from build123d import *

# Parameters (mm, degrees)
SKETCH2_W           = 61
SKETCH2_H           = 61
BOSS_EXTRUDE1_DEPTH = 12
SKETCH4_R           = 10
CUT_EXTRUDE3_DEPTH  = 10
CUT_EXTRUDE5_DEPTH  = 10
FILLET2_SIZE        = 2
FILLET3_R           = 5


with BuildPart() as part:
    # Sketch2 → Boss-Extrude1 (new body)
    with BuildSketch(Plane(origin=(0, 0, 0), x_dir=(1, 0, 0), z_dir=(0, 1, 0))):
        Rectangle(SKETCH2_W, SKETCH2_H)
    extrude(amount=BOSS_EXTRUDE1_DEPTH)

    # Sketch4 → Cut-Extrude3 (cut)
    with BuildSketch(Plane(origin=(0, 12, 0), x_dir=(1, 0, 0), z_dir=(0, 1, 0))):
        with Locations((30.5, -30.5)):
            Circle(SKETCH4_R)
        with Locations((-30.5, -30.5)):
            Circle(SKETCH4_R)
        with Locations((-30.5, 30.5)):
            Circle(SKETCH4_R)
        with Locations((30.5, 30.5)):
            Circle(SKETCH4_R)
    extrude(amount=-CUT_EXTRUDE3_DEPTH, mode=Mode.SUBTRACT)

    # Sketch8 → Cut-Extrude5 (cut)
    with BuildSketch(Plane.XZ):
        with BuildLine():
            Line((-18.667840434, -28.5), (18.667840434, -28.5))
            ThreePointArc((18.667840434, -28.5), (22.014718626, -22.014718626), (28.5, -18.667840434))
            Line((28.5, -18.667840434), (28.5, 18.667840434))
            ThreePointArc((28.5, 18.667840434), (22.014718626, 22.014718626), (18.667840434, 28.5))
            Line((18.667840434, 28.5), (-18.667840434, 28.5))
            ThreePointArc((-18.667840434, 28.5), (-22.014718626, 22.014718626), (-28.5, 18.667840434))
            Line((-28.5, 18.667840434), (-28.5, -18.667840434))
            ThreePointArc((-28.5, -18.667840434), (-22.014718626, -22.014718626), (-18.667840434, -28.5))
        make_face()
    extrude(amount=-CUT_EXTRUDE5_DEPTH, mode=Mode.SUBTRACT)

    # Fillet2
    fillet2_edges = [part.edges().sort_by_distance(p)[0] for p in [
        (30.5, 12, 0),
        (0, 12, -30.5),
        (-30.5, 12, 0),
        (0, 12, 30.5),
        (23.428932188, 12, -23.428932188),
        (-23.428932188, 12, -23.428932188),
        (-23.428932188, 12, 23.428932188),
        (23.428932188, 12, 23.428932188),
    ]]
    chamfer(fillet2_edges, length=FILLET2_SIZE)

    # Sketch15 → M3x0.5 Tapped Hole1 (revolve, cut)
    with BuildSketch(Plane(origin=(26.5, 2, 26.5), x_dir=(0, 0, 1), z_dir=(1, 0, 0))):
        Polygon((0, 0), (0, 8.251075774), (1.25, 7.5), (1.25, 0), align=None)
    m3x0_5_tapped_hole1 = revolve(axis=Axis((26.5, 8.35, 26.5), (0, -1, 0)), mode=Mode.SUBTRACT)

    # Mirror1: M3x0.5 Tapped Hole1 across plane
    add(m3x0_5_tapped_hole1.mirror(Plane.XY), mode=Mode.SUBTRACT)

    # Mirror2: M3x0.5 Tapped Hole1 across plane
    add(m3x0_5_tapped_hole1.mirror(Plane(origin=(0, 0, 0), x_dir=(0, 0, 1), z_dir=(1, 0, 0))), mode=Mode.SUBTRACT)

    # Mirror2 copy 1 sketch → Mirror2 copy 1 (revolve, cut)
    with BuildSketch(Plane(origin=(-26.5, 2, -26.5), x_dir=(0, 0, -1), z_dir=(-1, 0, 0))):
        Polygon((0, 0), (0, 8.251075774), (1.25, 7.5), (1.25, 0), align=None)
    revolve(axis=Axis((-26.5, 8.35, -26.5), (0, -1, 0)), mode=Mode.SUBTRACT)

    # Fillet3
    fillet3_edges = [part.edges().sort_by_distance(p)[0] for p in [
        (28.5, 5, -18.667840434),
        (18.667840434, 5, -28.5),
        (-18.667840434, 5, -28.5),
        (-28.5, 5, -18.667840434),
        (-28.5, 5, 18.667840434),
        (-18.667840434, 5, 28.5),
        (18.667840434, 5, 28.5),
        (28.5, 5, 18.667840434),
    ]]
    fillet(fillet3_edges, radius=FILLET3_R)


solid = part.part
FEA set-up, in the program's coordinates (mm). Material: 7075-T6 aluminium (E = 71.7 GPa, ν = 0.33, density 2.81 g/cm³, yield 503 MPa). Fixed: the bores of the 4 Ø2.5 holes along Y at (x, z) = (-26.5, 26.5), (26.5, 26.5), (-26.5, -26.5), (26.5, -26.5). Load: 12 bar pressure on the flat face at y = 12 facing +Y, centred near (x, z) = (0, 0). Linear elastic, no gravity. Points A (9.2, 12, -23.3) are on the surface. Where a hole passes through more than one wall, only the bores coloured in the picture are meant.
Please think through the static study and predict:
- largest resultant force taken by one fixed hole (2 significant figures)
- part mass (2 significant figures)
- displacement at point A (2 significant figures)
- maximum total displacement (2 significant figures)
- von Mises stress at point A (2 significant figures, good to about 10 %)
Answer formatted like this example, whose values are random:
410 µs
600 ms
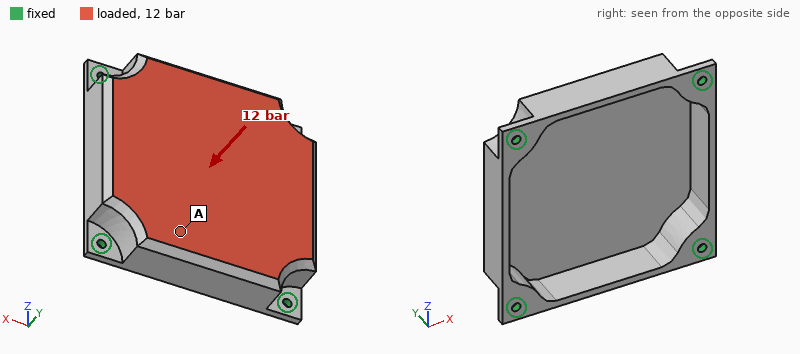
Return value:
1.1 kN
32 g
0.14 mm
0.53 mm
93 MPa
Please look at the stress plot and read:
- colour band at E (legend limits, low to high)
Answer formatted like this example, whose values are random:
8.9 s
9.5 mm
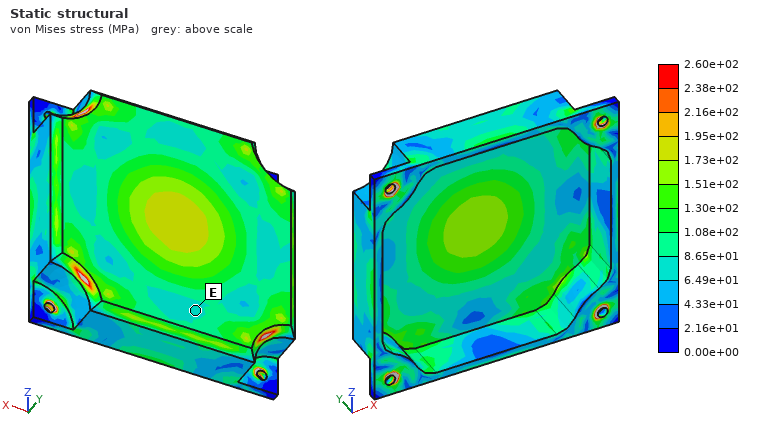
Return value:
6.49e+01 to 8.65e+01 MPa
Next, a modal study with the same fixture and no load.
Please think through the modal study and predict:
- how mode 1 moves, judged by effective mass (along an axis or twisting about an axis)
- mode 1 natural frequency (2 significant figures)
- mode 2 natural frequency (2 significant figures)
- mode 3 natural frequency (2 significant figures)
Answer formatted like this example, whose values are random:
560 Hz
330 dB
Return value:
along Y
4000 Hz
7900 Hz
7900 Hz
